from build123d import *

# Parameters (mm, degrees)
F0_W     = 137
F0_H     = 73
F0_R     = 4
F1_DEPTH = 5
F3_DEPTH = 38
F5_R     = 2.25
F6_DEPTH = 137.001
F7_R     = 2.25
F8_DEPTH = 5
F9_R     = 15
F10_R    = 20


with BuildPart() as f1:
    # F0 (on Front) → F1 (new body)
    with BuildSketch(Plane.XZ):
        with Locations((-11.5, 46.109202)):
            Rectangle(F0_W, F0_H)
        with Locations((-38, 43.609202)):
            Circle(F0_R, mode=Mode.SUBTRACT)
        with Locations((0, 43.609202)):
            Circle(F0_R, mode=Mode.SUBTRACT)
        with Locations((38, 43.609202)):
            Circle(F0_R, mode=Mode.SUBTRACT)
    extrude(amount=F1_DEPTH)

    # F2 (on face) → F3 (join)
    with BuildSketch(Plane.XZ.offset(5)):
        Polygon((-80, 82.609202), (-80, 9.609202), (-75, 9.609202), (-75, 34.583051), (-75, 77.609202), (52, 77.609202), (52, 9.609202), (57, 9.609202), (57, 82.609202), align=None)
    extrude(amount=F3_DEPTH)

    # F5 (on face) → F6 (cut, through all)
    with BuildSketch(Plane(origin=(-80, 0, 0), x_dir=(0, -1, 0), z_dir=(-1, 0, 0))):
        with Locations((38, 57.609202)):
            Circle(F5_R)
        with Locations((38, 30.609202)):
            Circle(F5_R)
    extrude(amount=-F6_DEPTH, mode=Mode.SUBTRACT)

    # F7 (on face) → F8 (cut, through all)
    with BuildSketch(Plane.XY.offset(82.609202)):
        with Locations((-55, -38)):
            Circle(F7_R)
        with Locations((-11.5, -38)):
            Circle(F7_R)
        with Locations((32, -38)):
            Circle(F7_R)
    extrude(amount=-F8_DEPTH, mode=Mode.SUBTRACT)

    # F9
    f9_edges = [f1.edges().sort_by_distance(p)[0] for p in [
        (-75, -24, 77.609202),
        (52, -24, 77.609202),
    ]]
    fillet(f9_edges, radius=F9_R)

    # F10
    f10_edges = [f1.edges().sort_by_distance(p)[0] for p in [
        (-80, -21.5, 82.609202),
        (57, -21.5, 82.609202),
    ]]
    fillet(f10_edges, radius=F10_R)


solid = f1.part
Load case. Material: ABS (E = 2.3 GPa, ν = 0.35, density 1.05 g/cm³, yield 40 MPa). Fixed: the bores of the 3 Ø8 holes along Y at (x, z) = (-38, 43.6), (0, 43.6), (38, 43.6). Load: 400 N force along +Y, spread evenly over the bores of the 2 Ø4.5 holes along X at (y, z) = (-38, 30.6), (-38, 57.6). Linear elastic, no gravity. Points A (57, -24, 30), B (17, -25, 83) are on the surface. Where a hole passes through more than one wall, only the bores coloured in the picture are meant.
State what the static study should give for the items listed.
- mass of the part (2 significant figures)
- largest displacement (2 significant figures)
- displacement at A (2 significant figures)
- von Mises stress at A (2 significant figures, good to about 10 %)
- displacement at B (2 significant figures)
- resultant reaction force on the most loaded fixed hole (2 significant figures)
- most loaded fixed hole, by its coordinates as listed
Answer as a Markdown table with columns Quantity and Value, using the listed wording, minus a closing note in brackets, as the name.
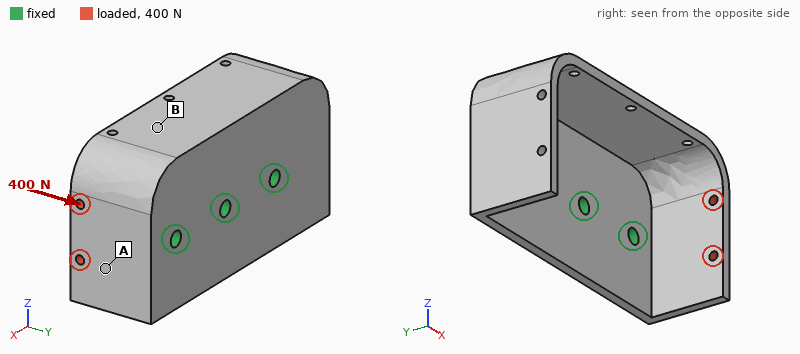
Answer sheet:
| Quantity | Value |
|---|---|
| mass of the part | 100 g |
| largest displacement | 0.96 mm |
| displacement at A | 0.61 mm |
| von Mises stress at A | 3.1 MPa |
| displacement at B | 0.16 mm |
| resultant reaction force on the most loaded fixed hole | 440 N |
| most loaded fixed hole, by its coordinates as listed | (38, 43.6) |
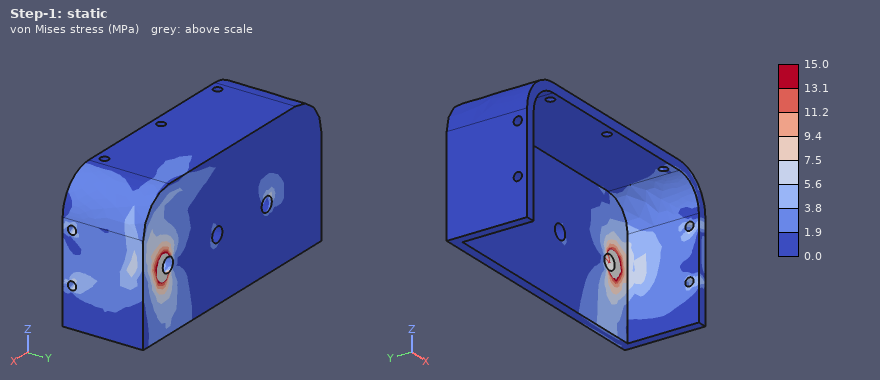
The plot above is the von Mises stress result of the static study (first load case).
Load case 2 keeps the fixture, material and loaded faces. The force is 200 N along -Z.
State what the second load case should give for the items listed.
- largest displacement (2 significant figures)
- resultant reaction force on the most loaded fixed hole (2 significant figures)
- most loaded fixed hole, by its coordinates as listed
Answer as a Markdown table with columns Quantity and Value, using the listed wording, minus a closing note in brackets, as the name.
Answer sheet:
| Quantity | Value |
|---|---|
| largest displacement | 1.8 mm |
| resultant reaction force on the most loaded fixed hole | 240 N |
| most loaded fixed hole, by its coordinates as listed | (38, 43.6) |
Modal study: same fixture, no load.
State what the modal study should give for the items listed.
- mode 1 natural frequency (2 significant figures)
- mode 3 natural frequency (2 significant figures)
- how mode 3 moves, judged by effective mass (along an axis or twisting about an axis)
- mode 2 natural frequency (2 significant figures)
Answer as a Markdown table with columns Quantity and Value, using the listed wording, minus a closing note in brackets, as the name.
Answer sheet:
| Quantity | Value |
|---|---|
| mode 1 natural frequency | 300 Hz |
| mode 3 natural frequency | 470 Hz |
| how mode 3 moves, judged by effective mass | along Y |
| mode 2 natural frequency | 380 Hz |
